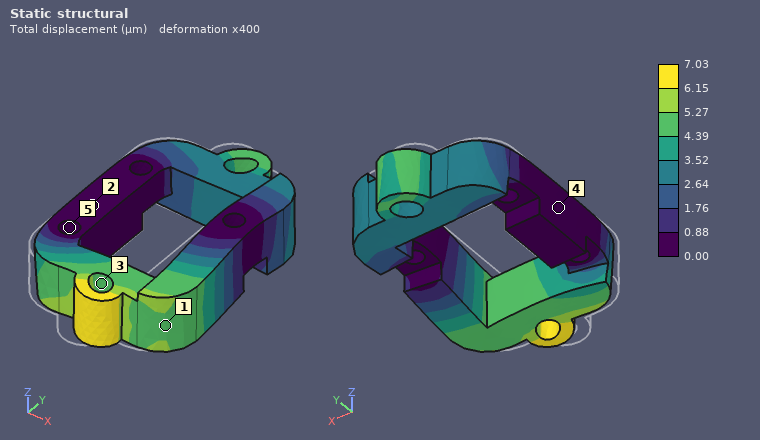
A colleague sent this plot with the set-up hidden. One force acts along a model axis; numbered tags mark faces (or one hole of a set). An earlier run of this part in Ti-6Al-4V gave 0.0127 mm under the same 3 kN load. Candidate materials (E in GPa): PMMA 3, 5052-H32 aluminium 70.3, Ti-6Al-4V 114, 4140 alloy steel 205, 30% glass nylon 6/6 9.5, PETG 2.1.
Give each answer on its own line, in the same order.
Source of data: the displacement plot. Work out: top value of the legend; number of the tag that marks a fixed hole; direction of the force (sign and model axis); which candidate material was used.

7.03 µm
5
+X
4140 alloy steel
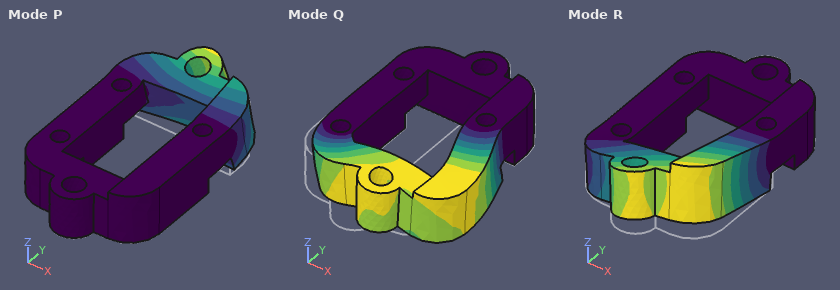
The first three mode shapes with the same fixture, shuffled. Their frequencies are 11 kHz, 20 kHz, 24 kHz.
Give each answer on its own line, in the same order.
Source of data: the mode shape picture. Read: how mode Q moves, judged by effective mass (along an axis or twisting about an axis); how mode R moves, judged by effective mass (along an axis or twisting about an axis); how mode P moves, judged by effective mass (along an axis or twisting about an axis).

along X
along Z
along Z
